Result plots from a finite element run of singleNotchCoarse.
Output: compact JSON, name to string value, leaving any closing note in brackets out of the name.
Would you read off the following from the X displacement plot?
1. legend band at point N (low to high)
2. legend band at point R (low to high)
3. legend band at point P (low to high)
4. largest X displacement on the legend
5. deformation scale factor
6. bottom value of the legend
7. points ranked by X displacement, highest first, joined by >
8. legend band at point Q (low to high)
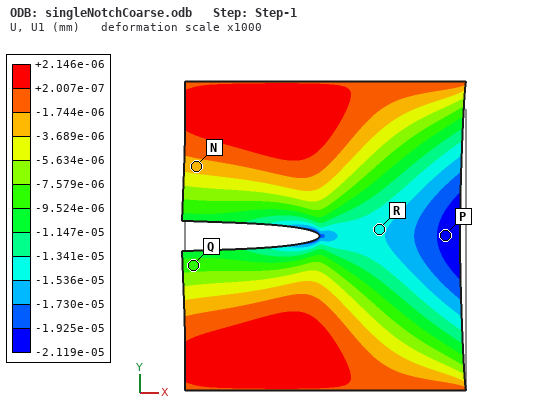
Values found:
{"legend band at point N": "-3.689e-06 to -1.744e-06 mm", "legend band at point R": "-1.536e-05 to -1.341e-05 mm", "legend band at point P": "-2.119e-05 to -1.925e-05 mm", "largest X displacement on the legend": "+2.146e-06 mm", "deformation scale factor": "1000", "bottom value of the legend": "-2.119e-05 mm", "points ranked by X displacement, highest first, joined by >": "N > Q > R > P", "legend band at point Q": "-9.524e-06 to -7.579e-06 mm"}
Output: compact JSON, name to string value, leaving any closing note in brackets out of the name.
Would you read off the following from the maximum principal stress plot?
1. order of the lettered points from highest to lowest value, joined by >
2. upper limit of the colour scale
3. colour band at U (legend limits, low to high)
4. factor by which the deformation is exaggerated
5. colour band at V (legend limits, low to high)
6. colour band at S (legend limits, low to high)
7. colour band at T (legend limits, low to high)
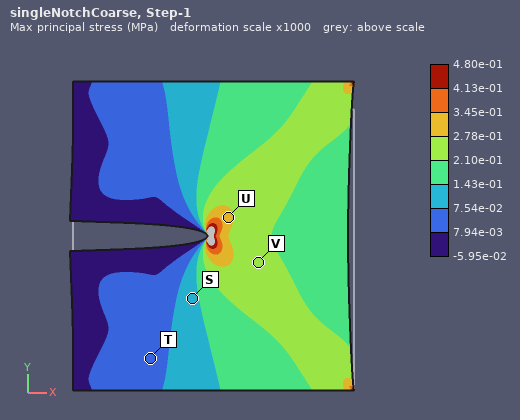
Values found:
{"order of the lettered points from highest to lowest value, joined by >": "U > V > S > T", "upper limit of the colour scale": "4.80e-01 MPa", "colour band at U": "2.78e-01 to 3.45e-01 MPa", "factor by which the deformation is exaggerated": "1000", "colour band at V": "2.10e-01 to 2.78e-01 MPa", "colour band at S": "7.54e-02 to 1.43e-01 MPa", "colour band at T": "7.94e-03 to 7.54e-02 MPa"}
